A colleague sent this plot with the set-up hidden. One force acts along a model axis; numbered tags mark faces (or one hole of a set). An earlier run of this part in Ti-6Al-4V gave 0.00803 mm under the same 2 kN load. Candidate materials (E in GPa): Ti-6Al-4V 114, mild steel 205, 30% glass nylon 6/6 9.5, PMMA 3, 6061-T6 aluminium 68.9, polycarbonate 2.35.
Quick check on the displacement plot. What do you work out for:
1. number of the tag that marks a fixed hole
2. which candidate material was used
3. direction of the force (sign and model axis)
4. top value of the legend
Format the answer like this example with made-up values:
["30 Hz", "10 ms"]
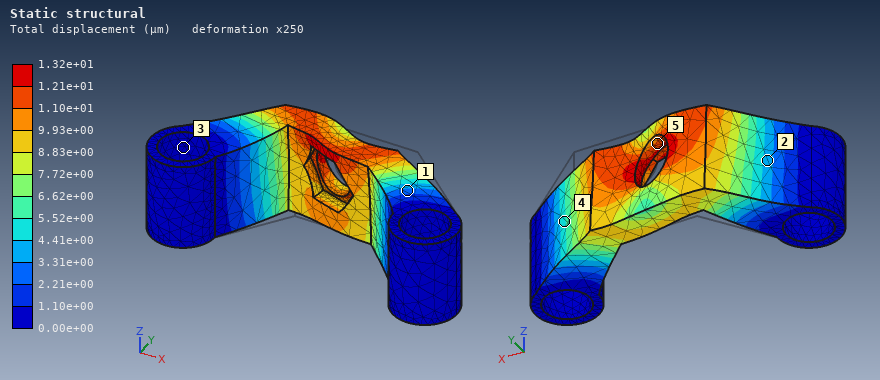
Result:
["3", "6061-T6 aluminium", "-X", "1.32e+01 µm"]
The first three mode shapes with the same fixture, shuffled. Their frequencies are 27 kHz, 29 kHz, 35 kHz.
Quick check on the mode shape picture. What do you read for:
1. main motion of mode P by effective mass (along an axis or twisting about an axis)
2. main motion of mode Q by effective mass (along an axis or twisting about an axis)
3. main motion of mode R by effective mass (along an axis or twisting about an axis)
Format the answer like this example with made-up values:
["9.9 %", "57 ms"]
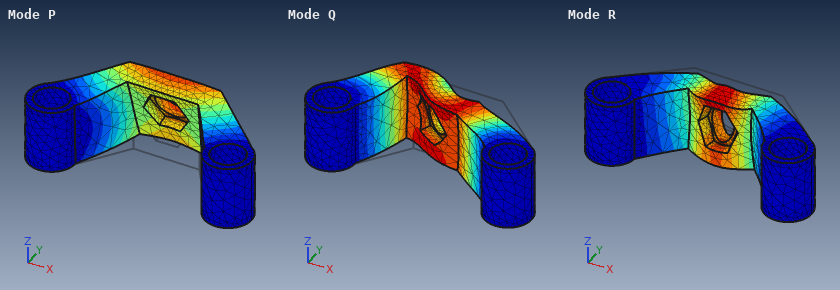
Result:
["along Z", "along X", "along Y"]
